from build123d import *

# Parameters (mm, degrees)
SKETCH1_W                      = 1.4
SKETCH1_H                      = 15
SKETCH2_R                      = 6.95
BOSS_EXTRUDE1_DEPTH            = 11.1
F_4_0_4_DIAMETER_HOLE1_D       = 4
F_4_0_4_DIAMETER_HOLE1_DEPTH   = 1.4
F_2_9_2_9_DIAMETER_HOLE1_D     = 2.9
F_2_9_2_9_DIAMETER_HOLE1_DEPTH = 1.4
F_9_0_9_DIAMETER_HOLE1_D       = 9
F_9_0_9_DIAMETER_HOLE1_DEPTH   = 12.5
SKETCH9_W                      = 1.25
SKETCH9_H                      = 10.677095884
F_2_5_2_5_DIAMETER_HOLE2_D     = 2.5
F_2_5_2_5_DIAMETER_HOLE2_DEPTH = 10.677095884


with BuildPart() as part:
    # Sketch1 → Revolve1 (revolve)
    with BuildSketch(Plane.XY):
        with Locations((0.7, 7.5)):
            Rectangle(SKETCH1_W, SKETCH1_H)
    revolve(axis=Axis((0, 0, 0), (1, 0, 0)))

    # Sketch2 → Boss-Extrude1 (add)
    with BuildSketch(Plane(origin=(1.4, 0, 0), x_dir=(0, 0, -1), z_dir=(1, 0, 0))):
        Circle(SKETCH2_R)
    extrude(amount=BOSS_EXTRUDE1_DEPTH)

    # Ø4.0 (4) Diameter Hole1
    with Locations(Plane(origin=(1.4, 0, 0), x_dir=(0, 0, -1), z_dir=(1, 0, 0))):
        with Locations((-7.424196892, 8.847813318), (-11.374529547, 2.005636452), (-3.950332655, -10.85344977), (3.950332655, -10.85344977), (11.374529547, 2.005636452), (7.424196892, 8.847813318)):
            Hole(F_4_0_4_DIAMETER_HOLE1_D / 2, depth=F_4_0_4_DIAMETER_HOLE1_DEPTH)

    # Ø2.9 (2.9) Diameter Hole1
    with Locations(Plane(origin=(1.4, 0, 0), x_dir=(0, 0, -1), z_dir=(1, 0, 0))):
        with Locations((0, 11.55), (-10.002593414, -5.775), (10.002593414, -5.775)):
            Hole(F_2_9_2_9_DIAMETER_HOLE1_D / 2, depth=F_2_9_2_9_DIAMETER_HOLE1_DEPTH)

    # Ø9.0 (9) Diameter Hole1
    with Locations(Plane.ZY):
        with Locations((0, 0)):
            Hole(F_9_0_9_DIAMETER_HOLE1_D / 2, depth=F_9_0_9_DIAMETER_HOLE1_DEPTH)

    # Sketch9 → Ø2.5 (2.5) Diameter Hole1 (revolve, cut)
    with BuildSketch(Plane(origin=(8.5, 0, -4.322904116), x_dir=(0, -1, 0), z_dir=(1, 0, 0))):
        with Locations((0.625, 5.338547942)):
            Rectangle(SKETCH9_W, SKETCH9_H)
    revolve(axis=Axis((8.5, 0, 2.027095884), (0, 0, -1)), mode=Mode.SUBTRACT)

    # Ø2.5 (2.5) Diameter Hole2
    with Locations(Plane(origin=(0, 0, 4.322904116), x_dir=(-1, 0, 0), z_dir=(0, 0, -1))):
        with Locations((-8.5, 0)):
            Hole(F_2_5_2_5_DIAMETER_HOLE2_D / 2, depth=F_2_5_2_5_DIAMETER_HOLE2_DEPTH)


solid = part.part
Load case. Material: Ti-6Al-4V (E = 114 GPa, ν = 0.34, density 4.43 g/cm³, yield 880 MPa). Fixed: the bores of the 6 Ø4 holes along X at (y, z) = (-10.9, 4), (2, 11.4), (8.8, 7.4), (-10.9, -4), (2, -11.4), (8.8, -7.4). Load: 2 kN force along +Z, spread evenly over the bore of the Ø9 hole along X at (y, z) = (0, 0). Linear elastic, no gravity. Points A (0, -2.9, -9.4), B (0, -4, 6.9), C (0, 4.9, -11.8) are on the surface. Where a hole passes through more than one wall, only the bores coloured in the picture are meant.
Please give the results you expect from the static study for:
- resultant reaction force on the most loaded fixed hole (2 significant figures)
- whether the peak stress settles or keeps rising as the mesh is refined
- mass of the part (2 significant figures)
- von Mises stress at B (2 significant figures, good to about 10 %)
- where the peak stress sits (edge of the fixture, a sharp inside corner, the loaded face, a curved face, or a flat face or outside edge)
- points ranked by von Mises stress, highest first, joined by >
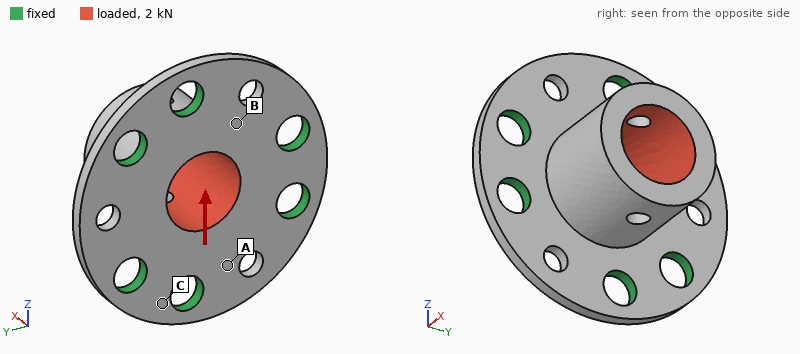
670 N
keeps rising
7.6 g
71 MPa
edge of the fixture
B > A > C
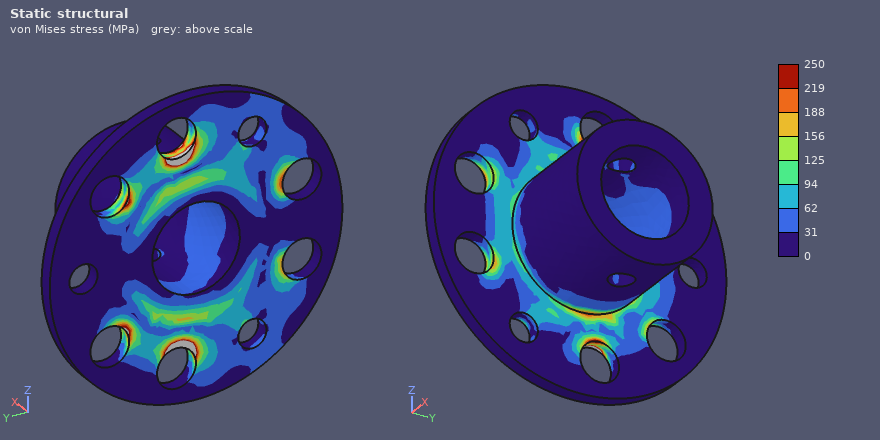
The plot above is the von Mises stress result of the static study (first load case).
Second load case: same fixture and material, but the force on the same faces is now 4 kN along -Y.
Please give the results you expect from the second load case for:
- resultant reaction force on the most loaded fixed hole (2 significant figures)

1.2 kN
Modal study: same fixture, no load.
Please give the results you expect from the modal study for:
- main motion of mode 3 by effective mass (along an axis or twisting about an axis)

along X
